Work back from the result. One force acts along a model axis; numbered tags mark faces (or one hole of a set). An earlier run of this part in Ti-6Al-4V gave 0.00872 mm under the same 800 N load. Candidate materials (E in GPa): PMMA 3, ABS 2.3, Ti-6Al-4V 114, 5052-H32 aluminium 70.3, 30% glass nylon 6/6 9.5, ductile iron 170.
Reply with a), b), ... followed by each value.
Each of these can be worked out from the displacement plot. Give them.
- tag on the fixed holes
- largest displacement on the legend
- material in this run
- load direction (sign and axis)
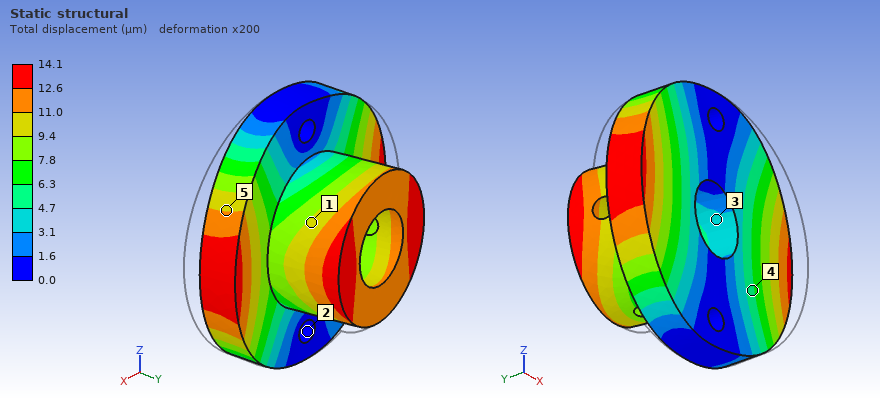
a) 2
b) 14.1 µm
c) 5052-H32 aluminium
d) -X
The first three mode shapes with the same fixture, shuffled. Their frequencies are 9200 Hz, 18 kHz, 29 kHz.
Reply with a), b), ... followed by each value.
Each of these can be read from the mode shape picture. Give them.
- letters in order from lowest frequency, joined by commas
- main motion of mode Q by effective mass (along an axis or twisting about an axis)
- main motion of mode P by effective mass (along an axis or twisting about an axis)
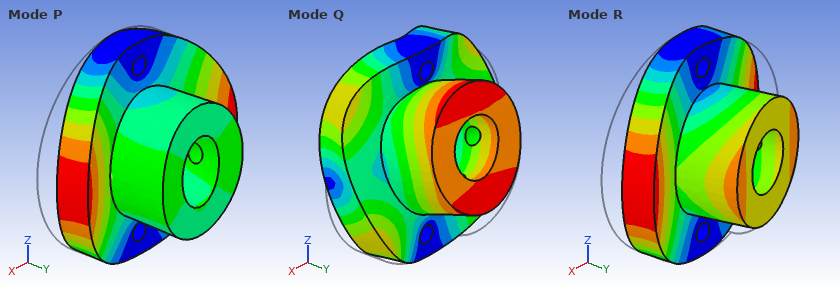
a) R, P, Q
b) along Z
c) along Y
